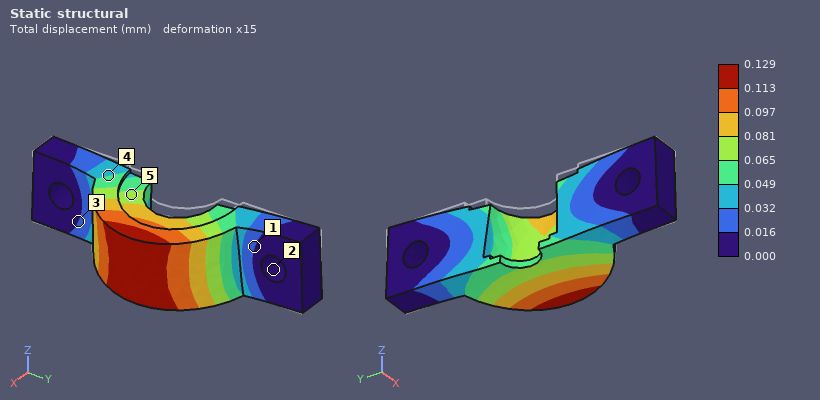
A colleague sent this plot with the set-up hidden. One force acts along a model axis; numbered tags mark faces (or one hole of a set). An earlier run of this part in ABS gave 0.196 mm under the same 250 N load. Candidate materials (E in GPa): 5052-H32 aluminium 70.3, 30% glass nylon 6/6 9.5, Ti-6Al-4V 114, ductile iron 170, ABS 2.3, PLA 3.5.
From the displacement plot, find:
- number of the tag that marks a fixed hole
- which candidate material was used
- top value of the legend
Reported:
2
PLA
0.129 mm
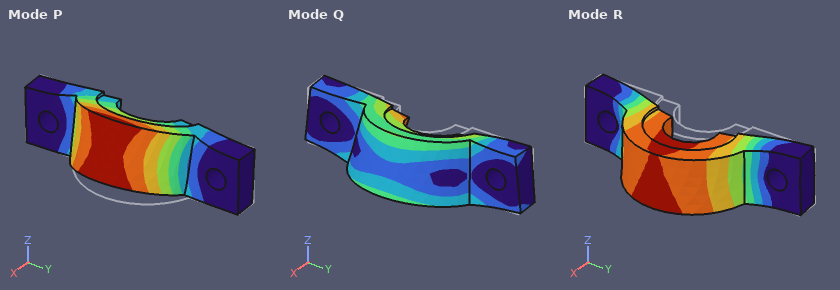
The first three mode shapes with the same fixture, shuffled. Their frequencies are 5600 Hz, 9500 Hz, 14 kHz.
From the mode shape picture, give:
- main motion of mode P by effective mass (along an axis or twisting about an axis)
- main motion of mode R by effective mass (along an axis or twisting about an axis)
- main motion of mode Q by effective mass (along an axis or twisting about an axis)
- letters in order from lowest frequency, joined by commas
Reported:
along Z
along X
along Z
P, R, Q
